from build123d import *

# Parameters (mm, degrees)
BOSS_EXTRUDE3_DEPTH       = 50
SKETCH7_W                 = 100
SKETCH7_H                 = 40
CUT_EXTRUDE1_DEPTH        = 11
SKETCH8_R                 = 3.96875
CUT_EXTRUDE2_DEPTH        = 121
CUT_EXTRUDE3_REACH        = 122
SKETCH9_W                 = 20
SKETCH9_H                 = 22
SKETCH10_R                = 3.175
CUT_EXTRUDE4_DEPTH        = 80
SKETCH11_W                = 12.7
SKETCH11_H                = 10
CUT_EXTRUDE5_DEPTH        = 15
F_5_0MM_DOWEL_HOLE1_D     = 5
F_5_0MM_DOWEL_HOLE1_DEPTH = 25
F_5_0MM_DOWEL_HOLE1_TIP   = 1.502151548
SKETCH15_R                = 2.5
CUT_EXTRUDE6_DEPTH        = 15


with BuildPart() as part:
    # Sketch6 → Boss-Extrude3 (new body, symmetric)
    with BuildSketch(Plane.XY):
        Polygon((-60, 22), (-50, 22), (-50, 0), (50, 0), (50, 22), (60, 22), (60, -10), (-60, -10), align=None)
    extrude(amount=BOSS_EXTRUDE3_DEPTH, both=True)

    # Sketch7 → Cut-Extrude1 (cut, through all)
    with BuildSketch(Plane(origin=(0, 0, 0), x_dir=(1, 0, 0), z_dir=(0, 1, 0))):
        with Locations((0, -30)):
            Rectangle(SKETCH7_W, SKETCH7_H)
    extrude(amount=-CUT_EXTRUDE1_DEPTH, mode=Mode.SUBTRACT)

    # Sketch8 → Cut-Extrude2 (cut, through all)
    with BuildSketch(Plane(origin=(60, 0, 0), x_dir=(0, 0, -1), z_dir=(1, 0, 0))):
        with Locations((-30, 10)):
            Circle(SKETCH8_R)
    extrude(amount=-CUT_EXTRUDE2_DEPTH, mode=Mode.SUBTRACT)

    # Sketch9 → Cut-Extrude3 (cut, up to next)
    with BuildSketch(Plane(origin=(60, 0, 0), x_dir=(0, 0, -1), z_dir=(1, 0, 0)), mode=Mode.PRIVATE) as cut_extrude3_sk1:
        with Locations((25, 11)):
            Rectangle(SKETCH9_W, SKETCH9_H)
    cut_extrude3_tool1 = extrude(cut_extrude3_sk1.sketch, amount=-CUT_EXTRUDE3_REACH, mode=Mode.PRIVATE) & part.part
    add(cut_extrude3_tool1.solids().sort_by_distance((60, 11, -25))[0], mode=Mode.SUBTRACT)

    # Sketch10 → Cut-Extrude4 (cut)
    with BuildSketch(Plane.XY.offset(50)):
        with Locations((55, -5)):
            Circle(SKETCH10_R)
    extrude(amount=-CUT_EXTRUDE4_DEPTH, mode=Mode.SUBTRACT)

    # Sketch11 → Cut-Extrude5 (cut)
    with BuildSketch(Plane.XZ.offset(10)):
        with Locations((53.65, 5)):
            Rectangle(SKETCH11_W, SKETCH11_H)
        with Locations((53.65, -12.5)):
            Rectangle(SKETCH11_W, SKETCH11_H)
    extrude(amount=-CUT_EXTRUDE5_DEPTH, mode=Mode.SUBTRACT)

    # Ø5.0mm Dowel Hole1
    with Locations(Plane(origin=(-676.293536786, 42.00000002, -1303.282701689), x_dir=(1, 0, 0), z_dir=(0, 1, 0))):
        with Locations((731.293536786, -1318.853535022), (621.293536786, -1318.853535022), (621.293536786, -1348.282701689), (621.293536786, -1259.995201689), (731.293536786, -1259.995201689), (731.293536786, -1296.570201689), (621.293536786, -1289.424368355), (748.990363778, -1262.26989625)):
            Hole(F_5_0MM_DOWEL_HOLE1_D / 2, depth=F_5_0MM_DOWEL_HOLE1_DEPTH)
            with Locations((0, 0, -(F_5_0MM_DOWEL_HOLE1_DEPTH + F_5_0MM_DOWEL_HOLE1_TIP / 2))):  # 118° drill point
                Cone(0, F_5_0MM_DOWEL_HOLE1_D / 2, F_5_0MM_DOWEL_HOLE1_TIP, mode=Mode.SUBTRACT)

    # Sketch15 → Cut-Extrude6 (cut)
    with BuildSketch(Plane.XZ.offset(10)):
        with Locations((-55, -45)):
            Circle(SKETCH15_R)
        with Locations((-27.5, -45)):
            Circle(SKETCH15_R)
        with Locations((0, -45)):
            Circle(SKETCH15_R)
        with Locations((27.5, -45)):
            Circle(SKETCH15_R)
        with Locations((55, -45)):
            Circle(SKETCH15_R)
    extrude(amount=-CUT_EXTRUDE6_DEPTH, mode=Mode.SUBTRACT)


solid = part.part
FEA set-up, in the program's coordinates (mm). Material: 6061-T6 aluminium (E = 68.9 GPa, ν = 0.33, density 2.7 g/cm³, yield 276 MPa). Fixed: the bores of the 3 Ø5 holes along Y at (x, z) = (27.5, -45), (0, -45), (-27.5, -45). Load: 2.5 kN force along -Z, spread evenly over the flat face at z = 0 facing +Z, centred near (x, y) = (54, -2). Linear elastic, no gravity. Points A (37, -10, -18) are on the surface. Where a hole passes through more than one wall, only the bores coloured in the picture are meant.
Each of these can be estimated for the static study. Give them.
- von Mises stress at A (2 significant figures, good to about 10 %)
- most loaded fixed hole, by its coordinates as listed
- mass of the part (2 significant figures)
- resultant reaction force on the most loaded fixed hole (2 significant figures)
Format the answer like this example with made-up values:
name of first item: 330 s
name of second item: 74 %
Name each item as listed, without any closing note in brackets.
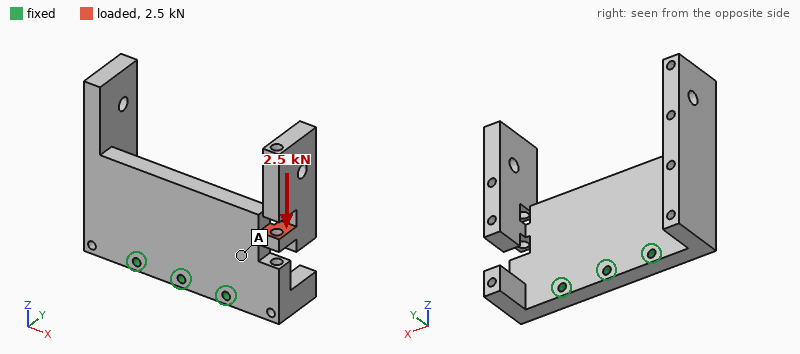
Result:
von Mises stress at A: 13 MPa
most loaded fixed hole, by its coordinates as listed: (27.5, -45)
mass of the part: 300 g
resultant reaction force on the most loaded fixed hole: 3.4 kN
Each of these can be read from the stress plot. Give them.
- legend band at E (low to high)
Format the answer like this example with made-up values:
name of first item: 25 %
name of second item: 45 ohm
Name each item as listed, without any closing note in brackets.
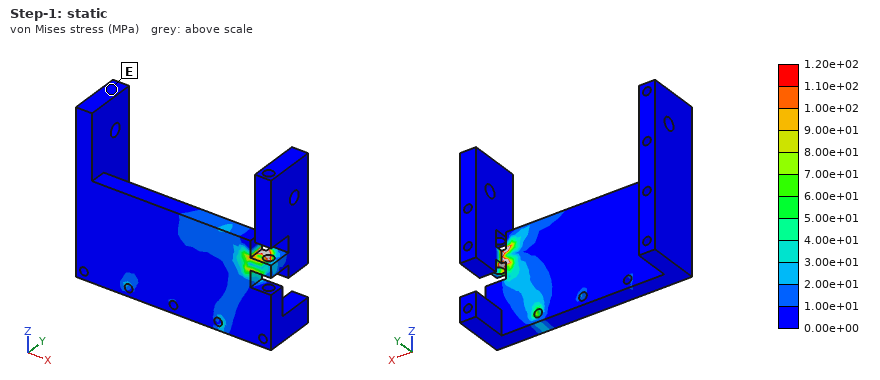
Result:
legend band at E: 0.00e+00 to 1.00e+01 MPa
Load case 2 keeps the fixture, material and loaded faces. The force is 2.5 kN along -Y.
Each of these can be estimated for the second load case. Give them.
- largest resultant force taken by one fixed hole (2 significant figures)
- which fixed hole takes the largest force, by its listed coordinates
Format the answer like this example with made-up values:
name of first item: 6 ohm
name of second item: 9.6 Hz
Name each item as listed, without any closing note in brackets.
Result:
largest resultant force taken by one fixed hole: 3.2 kN
which fixed hole takes the largest force, by its listed coordinates: (27.5, -45)
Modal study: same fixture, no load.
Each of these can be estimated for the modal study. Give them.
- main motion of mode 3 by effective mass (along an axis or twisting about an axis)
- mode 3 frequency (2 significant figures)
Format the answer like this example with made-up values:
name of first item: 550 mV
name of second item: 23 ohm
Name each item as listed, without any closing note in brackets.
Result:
main motion of mode 3 by effective mass: along Y
mode 3 frequency: 1000 Hz
